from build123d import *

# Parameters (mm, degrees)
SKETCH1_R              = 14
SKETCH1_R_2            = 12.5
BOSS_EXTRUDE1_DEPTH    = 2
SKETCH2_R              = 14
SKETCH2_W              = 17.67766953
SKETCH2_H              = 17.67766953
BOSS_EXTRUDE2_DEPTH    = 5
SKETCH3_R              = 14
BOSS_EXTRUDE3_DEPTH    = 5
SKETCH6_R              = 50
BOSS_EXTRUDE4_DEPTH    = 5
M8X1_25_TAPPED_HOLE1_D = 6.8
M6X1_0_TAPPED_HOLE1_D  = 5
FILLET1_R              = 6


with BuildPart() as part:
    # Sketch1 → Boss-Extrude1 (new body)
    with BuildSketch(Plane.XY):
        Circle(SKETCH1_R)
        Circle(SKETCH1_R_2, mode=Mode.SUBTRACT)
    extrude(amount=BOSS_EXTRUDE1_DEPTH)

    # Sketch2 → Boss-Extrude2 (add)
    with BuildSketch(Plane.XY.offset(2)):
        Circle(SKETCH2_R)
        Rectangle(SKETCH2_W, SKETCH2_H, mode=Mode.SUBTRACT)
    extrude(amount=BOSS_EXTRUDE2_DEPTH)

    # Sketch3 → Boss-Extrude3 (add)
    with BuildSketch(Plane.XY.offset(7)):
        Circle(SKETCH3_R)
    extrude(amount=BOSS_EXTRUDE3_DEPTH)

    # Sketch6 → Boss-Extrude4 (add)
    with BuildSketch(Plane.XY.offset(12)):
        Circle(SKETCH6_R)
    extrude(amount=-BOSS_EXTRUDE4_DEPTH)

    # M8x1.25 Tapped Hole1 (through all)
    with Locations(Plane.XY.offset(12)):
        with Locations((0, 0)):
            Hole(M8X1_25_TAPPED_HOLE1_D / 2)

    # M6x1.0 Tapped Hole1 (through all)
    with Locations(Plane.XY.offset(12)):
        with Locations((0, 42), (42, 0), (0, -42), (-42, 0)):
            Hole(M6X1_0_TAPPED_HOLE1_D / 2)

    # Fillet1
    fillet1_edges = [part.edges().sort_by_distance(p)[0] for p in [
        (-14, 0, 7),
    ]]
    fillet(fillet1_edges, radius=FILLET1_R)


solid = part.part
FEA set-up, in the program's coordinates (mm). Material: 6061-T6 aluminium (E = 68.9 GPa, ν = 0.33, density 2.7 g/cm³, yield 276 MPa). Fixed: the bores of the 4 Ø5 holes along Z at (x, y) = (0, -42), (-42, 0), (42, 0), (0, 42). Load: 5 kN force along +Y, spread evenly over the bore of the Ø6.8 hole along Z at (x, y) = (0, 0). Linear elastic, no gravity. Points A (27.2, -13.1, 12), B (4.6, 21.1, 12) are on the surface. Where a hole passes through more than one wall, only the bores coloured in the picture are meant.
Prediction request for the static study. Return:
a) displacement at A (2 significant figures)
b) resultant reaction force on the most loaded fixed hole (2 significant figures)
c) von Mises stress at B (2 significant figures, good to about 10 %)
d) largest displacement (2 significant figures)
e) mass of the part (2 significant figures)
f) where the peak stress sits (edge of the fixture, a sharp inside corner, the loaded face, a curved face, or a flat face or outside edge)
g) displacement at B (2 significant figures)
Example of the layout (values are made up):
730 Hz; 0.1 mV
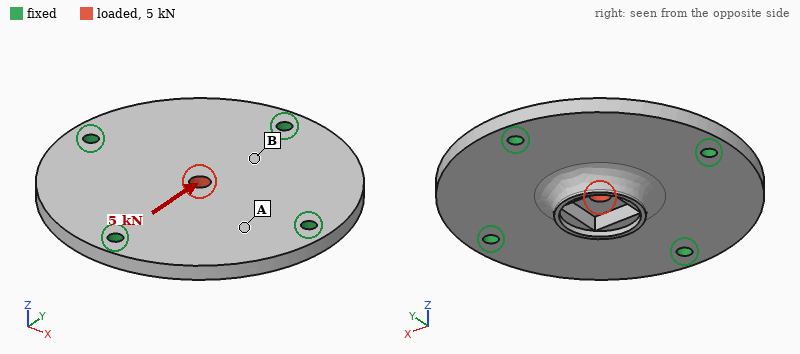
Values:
3.7 µm; 1.6 kN; 16 MPa; 13 µm; 110 g; the loaded face; 5.4 µm
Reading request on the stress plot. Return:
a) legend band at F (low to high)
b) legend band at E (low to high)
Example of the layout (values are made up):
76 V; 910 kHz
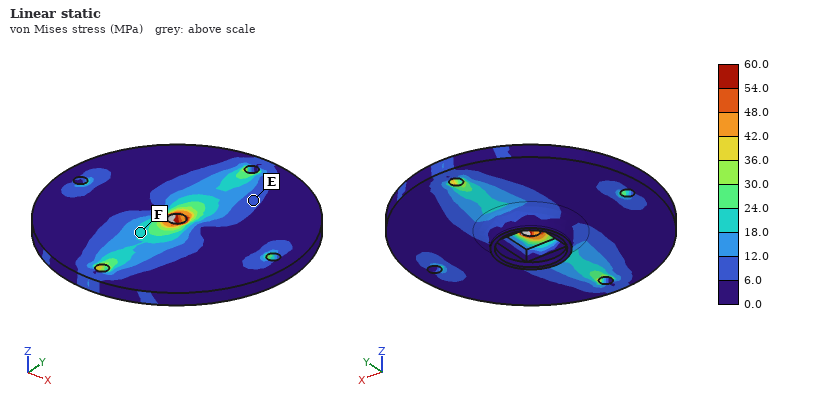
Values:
18.0 to 24.0 MPa; 6.0 to 12.0 MPa
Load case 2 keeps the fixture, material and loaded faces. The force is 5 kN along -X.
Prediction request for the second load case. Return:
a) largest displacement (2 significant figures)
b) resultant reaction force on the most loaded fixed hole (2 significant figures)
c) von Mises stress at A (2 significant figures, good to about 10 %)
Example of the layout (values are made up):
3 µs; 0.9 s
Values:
13 µm; 1.6 kN; 8.0 MPa
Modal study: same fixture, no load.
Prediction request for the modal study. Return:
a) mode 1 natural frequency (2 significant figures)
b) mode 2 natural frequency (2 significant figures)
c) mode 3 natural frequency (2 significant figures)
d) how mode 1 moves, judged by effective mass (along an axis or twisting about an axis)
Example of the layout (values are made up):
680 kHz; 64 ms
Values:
5300 Hz; 5800 Hz; 6000 Hz; along Z
